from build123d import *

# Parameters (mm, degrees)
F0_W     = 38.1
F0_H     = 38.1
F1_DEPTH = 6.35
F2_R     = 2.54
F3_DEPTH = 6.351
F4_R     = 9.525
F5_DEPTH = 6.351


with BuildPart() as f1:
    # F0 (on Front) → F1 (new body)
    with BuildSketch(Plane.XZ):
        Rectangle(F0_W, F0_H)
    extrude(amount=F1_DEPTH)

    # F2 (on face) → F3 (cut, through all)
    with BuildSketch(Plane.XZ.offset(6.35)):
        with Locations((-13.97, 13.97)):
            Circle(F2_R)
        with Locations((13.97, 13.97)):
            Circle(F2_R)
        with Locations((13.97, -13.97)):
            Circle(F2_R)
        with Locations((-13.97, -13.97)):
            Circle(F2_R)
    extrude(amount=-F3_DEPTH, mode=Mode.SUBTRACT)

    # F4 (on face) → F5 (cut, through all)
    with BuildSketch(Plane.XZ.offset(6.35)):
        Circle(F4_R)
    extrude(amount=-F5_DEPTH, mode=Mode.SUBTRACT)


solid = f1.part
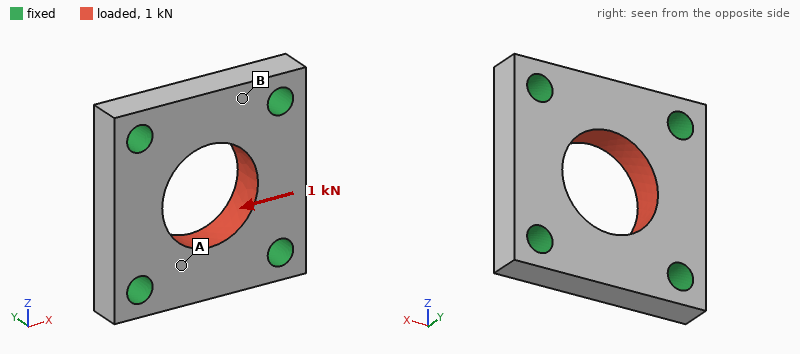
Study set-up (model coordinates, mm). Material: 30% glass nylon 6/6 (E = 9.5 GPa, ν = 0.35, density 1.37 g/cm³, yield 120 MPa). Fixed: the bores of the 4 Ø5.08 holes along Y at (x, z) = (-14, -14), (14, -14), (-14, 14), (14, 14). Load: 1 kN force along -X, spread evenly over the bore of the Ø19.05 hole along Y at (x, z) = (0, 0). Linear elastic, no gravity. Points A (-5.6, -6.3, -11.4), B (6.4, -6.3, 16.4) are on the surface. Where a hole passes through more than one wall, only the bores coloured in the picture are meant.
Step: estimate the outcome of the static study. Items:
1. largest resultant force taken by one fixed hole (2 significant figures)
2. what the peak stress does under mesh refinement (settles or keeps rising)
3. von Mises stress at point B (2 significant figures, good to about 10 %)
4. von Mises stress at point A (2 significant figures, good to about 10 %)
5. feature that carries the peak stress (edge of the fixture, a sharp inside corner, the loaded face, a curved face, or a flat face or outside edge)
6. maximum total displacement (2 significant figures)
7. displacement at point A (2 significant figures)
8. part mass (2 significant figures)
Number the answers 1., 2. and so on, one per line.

1. 260 N
2. keeps rising
3. 1.6 MPa
4. 3.8 MPa
5. edge of the fixture
6. 8.7 µm
7. 2.7 µm
8. 9.4 g
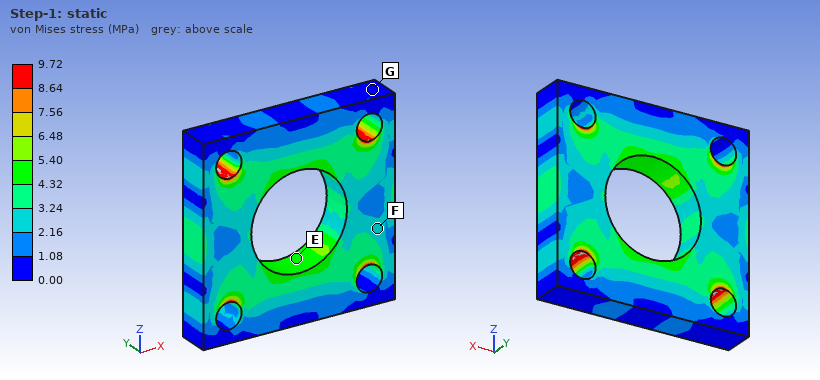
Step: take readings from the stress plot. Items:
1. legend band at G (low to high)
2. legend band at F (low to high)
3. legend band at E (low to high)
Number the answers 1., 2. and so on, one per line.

1. 0.00 to 1.08 MPa
2. 2.16 to 3.24 MPa
3. 4.32 to 5.40 MPa
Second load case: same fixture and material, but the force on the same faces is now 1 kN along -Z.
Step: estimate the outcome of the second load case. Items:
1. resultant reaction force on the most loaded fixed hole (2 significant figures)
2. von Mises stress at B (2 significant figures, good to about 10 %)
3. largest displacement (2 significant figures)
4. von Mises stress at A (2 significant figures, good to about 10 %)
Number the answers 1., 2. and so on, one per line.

1. 260 N
2. 2.6 MPa
3. 8.7 µm
4. 3.4 MPa
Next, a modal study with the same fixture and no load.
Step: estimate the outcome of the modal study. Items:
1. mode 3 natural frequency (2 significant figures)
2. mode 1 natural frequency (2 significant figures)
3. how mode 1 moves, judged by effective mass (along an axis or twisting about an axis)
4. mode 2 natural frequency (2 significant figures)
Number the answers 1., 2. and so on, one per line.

1. 21 kHz
2. 20 kHz
3. along Y
4. 20 kHz
